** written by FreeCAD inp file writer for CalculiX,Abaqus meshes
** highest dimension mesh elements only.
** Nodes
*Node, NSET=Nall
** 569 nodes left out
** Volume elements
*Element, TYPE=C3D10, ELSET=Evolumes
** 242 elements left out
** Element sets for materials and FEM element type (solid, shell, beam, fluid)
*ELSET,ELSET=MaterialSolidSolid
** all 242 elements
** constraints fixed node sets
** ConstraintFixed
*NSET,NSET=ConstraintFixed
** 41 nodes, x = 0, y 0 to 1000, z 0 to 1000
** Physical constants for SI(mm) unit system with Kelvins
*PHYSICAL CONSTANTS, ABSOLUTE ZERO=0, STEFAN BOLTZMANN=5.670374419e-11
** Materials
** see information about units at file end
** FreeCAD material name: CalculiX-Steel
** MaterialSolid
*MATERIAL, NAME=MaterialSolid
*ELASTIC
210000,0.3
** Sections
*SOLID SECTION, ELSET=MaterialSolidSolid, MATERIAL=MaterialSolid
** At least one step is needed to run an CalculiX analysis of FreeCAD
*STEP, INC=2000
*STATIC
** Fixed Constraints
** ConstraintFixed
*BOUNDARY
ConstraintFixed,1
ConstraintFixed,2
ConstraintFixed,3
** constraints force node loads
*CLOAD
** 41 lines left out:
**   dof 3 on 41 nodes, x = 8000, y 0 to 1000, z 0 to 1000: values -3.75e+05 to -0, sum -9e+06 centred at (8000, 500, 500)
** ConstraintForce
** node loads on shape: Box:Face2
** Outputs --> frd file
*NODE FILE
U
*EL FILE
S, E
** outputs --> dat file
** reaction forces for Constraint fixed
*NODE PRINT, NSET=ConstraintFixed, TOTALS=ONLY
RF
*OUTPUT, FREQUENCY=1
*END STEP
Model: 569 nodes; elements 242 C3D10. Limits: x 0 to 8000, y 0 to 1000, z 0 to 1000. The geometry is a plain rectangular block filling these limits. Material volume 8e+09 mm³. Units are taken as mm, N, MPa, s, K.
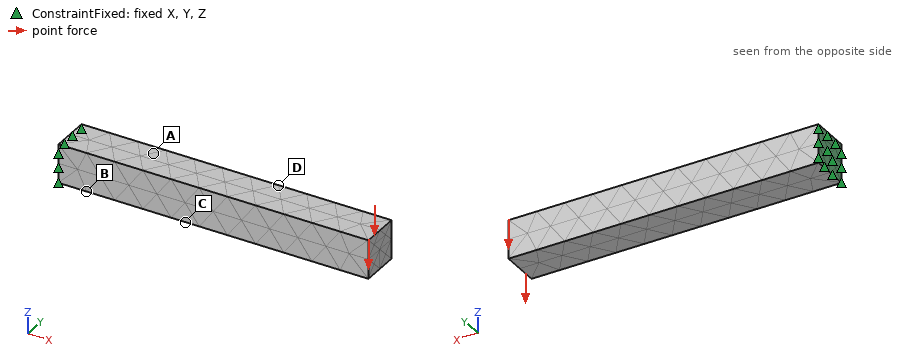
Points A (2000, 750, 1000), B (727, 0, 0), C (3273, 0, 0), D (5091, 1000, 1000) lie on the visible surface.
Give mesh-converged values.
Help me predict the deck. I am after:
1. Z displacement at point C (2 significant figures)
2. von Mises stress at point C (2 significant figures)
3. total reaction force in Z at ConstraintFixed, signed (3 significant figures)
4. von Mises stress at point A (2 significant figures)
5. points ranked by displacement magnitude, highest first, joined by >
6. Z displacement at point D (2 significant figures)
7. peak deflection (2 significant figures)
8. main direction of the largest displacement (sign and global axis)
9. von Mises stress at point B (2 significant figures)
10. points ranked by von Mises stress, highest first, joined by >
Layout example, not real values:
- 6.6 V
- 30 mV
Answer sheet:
- -19 mm
- 260 MPa
- 9.00e+06 N
- 320 MPa
- D > C > A > B
- -42 mm
- 88 mm
- -Z
- 390 MPa
- B > A > C > D
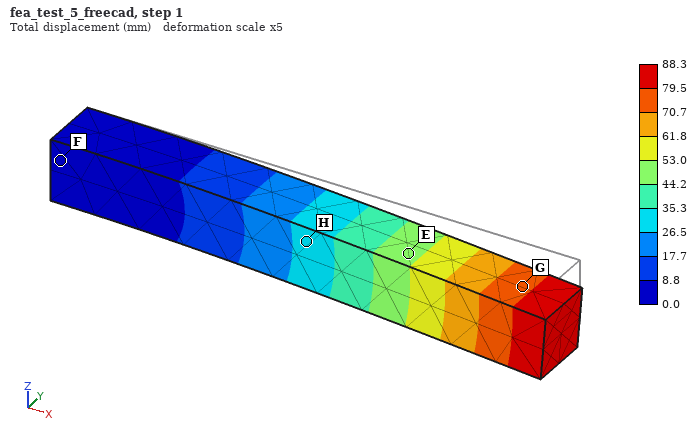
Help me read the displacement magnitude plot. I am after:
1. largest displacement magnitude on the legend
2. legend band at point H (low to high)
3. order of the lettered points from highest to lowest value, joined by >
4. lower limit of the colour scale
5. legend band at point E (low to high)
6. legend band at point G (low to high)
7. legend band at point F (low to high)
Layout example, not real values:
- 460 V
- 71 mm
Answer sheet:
- 88.3 mm
- 26.5 to 35.3 mm
- G > E > H > F
- 0.0 mm
- 44.2 to 53.0 mm
- 70.7 to 79.5 mm
- 0.0 to 8.8 mm
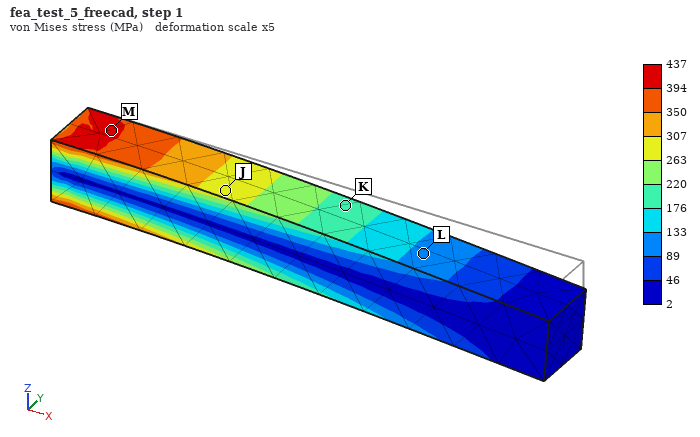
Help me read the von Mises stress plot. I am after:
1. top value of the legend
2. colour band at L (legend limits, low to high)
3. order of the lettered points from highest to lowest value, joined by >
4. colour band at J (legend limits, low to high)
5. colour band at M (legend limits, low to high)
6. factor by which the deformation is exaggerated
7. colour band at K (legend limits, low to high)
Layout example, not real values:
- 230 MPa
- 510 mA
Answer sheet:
- 437 MPa
- 89 to 133 MPa
- M > J > K > L
- 263 to 307 MPa
- 394 to 437 MPa
- 5
- 176 to 220 MPa
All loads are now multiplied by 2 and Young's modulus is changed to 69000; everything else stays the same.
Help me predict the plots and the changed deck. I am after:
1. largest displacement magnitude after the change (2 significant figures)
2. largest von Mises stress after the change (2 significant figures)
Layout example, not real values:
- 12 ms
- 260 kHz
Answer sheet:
- 540 mm
- 870 MPa
